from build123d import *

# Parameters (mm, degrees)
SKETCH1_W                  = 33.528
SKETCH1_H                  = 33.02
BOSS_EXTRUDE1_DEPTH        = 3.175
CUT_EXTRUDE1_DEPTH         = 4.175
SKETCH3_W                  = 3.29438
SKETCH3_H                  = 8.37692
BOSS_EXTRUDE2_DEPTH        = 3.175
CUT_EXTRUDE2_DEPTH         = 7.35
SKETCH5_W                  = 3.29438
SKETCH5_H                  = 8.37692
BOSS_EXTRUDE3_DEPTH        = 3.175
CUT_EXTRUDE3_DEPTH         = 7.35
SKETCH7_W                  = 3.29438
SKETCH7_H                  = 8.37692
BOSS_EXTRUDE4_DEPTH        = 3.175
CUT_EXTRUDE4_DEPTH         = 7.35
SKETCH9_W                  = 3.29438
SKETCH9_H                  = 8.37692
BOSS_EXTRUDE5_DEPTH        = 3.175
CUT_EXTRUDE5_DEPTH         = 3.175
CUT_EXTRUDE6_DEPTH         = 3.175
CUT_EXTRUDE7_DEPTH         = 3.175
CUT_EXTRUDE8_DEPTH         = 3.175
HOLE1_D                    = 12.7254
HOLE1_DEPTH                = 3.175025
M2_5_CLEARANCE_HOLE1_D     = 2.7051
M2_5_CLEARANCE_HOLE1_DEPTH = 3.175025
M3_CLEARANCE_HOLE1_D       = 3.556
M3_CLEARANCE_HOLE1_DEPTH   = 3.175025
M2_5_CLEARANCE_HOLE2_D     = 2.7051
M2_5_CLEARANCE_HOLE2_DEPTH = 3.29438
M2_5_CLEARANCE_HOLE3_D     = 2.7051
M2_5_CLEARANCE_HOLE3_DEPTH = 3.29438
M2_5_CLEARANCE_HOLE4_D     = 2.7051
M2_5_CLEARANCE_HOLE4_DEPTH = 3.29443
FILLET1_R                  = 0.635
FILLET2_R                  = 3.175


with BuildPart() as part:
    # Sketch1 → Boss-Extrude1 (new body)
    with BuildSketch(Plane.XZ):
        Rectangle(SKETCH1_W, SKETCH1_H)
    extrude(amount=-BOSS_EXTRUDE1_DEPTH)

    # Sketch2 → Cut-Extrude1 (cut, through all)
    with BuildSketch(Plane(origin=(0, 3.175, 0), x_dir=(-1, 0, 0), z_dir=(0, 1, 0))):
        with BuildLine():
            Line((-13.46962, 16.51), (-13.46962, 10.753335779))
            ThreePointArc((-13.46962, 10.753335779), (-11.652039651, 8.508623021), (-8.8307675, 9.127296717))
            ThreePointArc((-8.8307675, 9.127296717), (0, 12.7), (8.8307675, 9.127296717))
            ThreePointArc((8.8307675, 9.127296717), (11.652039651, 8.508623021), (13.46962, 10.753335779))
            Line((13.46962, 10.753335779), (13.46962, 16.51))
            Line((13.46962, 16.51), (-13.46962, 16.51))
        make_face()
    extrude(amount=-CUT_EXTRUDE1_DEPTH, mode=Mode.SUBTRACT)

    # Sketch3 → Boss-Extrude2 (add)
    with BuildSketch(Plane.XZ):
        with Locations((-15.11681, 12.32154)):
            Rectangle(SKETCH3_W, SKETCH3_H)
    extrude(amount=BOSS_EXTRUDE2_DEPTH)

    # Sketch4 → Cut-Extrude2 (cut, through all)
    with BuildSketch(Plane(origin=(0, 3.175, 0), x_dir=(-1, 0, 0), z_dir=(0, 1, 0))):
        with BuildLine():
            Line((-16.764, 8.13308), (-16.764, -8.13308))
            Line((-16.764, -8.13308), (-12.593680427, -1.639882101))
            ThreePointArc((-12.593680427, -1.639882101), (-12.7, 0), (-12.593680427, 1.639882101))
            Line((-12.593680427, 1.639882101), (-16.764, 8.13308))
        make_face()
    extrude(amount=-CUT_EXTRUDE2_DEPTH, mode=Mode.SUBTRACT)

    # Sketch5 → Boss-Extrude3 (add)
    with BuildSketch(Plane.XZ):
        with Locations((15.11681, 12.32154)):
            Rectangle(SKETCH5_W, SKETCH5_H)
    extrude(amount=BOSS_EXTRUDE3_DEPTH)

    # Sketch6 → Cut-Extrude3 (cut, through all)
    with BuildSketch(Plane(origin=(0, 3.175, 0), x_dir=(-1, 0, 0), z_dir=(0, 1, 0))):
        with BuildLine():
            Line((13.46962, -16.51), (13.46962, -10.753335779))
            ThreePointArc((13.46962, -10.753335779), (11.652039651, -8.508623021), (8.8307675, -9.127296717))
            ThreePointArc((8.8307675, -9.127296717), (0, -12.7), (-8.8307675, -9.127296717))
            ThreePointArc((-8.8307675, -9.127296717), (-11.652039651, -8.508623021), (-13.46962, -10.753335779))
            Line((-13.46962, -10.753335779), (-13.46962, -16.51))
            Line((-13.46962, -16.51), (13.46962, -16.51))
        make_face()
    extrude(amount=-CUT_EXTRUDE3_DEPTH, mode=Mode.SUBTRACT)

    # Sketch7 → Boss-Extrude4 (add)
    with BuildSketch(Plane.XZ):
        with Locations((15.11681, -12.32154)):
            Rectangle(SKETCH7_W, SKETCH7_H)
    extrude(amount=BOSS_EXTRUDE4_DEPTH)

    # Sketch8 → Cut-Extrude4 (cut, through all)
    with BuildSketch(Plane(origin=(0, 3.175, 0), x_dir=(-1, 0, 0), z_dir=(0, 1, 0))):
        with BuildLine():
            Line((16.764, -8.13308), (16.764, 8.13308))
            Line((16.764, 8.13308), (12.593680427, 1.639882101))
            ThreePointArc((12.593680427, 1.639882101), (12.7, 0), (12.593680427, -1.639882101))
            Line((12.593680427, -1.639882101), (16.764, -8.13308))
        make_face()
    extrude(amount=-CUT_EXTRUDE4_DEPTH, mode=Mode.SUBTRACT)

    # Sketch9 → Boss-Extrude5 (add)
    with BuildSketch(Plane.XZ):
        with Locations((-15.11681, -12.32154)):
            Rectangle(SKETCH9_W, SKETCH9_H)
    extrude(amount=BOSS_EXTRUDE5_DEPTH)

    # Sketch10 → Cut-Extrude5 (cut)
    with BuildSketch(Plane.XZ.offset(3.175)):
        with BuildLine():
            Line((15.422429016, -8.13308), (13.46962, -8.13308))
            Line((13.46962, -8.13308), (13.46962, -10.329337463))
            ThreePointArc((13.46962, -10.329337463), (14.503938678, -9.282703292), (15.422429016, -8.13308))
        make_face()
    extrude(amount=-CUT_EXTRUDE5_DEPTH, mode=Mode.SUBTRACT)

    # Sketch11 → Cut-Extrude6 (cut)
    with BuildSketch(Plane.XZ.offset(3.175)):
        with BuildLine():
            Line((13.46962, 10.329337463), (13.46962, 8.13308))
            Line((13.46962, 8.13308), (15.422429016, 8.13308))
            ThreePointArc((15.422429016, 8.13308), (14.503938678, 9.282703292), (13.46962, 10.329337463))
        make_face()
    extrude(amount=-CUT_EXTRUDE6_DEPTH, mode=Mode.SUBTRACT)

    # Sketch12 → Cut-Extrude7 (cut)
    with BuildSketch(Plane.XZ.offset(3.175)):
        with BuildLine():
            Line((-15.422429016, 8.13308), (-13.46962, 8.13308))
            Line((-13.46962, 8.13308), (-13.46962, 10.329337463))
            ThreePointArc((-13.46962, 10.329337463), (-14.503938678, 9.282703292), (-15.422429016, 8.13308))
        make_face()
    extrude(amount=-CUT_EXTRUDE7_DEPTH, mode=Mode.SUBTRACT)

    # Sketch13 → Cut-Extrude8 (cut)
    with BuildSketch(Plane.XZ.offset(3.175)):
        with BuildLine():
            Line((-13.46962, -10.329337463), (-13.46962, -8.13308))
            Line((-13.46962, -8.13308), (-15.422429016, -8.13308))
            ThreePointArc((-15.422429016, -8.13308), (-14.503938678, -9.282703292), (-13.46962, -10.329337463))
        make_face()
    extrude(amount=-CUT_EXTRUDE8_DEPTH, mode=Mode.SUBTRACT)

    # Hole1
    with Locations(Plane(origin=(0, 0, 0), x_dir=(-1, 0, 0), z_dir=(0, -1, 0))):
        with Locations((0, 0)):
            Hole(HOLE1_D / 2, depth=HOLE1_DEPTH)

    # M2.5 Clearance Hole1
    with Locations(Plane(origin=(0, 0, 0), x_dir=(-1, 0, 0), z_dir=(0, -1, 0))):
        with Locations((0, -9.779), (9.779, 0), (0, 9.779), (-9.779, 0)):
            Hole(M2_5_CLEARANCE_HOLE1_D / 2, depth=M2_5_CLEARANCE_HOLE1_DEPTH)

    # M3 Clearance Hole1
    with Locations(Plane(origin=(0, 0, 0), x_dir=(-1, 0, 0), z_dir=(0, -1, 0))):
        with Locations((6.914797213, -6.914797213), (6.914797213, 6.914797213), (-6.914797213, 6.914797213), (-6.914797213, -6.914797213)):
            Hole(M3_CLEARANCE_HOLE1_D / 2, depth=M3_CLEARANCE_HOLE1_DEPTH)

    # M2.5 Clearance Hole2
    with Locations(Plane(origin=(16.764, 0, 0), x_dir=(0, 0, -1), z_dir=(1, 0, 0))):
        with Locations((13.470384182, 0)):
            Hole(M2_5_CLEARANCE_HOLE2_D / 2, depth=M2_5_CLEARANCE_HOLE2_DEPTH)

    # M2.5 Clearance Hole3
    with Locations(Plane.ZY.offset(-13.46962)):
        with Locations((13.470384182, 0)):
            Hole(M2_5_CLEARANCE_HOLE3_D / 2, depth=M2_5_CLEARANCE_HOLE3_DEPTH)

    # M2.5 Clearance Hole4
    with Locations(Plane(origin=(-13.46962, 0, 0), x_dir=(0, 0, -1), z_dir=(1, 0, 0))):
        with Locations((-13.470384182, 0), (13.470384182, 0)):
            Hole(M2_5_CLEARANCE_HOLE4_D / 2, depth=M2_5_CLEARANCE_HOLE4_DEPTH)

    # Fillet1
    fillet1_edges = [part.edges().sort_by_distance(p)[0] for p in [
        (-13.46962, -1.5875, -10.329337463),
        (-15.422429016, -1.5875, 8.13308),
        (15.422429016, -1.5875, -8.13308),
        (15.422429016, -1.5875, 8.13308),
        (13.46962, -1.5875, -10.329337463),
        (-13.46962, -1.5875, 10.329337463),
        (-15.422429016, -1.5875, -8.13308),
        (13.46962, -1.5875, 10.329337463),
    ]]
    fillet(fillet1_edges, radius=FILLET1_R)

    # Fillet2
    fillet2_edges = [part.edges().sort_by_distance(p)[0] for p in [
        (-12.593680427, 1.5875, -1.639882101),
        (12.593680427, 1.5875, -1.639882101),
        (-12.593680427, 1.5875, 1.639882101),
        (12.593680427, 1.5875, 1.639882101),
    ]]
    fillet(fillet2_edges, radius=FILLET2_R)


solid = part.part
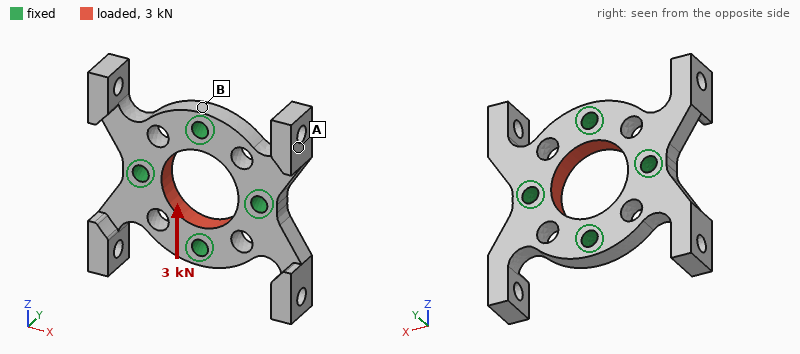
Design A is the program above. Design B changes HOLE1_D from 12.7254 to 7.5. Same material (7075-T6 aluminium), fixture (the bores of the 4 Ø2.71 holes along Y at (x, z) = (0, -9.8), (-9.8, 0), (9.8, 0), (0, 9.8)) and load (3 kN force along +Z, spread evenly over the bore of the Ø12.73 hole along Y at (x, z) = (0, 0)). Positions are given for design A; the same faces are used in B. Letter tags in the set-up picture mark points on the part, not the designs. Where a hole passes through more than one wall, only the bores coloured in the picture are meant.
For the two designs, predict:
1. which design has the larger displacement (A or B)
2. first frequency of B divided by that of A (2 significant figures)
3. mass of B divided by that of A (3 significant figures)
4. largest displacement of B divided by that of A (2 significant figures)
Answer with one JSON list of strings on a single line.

["B", "1.0", "1.14", "1.1"]
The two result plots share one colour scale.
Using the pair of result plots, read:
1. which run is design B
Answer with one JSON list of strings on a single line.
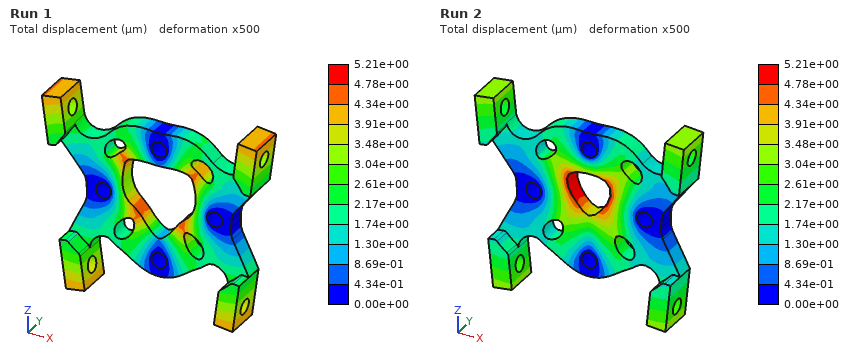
["Run 2"]
